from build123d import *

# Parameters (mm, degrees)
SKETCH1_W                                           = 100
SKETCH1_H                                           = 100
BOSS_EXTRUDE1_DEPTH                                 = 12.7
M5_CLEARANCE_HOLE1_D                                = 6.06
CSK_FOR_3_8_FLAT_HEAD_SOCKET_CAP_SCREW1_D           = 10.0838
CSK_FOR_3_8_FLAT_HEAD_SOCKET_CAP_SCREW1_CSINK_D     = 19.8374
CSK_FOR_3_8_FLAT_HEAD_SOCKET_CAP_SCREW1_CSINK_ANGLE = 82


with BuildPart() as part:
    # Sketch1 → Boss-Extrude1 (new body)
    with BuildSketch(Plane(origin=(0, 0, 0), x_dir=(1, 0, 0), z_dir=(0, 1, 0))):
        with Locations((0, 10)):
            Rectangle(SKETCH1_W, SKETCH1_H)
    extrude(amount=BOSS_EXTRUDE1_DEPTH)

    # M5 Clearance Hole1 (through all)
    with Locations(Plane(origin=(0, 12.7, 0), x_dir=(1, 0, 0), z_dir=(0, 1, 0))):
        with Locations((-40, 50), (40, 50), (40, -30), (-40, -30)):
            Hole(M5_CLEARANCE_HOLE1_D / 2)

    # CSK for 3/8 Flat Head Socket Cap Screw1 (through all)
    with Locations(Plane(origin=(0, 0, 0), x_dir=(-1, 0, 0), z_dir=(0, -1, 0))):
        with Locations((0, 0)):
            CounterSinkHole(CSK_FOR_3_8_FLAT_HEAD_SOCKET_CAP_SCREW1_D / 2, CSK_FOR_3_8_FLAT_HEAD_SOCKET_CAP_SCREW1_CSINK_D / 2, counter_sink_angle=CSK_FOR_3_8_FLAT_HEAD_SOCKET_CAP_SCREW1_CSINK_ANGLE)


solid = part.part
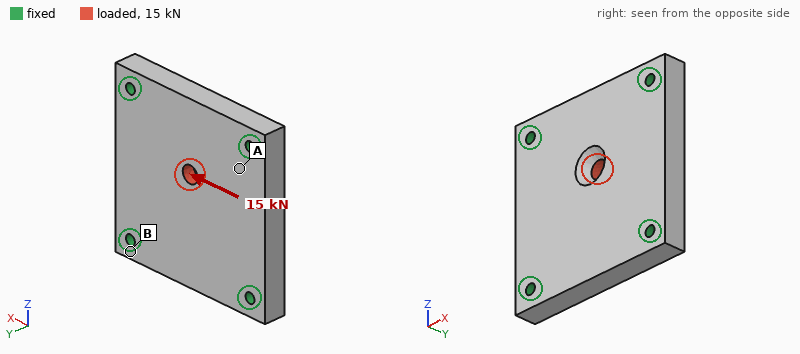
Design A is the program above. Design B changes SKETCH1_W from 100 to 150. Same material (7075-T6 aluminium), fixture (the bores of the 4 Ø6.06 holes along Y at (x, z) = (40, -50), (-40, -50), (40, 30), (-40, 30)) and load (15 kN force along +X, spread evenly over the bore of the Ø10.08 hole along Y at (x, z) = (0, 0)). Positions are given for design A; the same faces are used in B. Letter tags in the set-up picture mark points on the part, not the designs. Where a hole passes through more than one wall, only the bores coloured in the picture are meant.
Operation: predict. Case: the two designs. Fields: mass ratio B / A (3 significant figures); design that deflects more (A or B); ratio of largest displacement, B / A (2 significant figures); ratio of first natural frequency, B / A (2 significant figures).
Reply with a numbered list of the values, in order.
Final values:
1. 1.51
2. A
3. 0.90
4. 0.88
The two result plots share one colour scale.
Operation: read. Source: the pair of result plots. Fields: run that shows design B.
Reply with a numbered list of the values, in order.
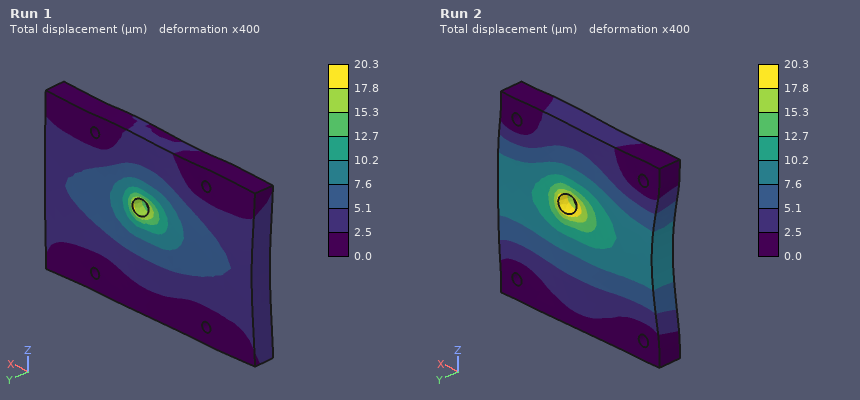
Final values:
1. Run 1
